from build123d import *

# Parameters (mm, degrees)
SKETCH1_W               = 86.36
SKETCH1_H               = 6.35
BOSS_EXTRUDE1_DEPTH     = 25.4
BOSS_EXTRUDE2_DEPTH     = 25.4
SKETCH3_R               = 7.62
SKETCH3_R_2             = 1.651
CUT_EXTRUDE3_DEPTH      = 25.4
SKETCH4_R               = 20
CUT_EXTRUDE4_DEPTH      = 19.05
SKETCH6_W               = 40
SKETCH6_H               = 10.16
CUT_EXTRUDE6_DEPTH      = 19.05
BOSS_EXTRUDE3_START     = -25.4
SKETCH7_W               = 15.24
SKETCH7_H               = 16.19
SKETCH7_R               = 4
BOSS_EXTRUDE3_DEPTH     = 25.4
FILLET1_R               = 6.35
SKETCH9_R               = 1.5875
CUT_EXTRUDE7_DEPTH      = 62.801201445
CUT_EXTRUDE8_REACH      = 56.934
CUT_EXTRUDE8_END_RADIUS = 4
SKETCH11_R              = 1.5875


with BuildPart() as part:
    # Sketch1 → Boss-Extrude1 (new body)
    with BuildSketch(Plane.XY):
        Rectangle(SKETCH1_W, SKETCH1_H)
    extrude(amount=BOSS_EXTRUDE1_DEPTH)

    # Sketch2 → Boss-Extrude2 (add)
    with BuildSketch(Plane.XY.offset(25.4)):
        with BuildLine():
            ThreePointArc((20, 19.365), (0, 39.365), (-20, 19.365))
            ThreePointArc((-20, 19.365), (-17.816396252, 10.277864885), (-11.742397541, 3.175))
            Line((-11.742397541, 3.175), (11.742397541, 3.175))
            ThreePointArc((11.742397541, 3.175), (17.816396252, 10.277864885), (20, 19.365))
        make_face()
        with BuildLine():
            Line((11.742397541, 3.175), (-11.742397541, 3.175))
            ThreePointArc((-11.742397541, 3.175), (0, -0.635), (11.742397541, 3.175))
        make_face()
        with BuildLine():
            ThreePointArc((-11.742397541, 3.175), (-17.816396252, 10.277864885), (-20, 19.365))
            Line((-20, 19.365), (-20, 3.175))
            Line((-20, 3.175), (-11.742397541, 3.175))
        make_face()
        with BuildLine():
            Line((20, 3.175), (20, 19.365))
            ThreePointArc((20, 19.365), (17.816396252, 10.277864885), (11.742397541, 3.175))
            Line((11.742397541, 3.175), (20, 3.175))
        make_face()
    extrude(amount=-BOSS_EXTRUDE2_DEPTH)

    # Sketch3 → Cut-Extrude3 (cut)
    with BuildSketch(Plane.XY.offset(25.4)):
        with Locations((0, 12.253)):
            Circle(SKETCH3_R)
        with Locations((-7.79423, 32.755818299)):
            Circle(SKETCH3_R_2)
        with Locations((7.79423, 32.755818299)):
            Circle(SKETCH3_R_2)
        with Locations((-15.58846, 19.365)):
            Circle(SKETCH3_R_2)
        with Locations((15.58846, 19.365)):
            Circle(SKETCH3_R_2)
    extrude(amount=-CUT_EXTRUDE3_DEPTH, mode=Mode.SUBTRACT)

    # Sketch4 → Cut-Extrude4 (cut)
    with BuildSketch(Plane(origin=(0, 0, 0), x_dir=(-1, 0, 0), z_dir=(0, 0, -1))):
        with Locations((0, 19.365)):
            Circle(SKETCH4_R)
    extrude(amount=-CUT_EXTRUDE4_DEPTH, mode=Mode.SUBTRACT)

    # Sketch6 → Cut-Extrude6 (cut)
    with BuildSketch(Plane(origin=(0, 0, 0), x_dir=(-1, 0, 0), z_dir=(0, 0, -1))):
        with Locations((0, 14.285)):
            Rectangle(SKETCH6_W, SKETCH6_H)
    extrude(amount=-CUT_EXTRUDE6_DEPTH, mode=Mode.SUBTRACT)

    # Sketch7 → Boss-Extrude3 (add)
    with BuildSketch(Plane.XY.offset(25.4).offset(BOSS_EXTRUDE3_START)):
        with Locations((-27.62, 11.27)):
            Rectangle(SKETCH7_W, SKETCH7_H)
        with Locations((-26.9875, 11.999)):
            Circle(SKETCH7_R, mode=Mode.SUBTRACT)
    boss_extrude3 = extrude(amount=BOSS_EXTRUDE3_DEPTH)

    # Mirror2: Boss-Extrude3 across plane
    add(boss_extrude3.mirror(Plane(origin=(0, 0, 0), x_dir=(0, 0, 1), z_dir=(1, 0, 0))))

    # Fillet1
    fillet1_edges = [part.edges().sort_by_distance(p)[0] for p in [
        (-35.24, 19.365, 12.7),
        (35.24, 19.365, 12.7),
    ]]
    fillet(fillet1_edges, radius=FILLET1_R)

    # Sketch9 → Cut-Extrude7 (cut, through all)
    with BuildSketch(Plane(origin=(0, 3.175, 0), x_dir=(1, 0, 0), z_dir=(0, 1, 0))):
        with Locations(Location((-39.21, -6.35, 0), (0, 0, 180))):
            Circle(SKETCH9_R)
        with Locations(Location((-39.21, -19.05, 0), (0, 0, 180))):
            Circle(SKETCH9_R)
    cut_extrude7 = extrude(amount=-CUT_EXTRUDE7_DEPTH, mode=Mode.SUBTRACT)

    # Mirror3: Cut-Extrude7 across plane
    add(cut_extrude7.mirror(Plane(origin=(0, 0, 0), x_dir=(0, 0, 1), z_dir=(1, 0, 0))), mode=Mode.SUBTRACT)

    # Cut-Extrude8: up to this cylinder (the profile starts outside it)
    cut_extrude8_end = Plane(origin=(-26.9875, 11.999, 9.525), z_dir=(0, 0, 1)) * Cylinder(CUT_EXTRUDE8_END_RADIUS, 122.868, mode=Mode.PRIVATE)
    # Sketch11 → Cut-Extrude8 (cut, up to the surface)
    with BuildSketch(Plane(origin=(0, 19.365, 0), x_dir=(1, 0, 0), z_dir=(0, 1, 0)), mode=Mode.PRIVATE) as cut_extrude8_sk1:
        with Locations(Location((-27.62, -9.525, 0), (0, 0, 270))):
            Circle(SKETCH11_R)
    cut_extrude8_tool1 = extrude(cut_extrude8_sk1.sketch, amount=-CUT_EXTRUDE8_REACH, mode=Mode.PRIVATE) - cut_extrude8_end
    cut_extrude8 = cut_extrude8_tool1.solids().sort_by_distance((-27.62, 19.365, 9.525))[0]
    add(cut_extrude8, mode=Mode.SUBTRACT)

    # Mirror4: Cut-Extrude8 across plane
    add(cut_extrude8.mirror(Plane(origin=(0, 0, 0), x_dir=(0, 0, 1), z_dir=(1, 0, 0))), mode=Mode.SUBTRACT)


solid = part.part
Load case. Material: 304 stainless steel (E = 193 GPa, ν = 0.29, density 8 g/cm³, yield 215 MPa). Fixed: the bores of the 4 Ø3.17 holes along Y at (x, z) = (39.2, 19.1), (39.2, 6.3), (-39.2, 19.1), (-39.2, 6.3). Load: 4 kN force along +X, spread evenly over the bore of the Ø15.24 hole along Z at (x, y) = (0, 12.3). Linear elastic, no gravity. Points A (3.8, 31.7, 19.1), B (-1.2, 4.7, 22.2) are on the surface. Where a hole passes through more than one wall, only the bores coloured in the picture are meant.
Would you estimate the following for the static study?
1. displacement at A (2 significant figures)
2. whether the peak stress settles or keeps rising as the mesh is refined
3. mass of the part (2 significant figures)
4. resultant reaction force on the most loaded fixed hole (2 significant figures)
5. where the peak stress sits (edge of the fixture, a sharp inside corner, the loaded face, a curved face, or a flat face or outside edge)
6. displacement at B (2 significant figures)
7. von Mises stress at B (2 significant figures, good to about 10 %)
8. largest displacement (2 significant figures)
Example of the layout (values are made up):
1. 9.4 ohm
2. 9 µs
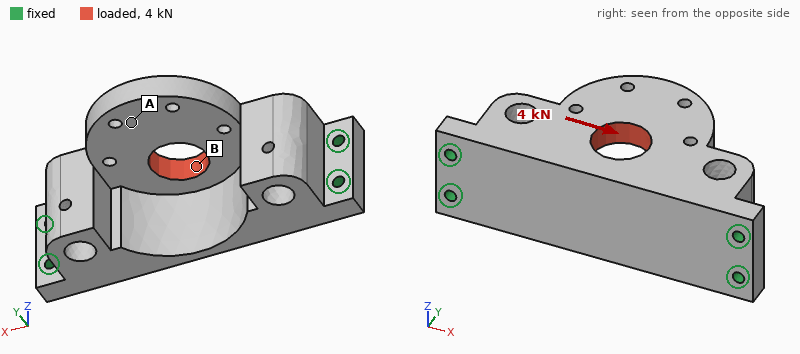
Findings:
1. 5.1 µm
2. keeps rising
3. 240 g
4. 1.4 kN
5. edge of the fixture
6. 2.4 µm
7. 26 MPa
8. 5.8 µm
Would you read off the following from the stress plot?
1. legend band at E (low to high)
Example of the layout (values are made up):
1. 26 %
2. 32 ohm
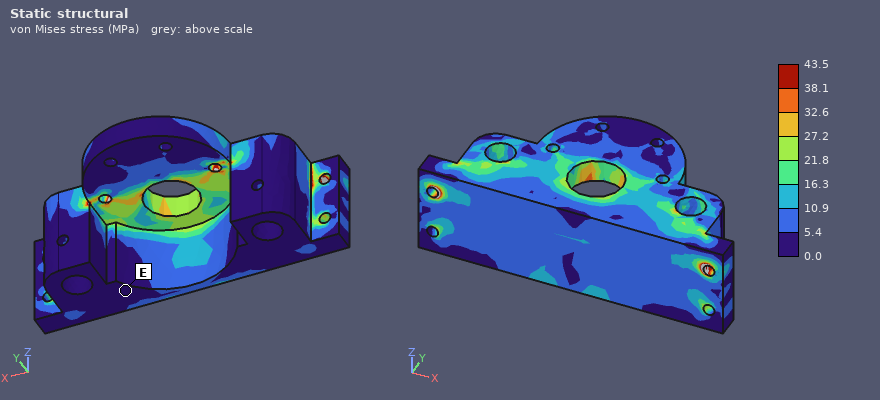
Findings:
1. 0.0 to 5.4 MPa
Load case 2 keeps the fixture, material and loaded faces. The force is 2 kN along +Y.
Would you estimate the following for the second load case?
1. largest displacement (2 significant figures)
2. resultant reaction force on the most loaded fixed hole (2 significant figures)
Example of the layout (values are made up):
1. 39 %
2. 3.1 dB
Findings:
1. 15 µm
2. 1.3 kN
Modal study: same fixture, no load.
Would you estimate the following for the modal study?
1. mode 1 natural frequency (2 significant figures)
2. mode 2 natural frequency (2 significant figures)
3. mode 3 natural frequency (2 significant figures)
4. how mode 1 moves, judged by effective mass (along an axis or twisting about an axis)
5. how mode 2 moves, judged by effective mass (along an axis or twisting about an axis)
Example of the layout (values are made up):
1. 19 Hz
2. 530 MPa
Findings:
1. 4600 Hz
2. 7200 Hz
3. 9600 Hz
4. along Z
5. along Y
